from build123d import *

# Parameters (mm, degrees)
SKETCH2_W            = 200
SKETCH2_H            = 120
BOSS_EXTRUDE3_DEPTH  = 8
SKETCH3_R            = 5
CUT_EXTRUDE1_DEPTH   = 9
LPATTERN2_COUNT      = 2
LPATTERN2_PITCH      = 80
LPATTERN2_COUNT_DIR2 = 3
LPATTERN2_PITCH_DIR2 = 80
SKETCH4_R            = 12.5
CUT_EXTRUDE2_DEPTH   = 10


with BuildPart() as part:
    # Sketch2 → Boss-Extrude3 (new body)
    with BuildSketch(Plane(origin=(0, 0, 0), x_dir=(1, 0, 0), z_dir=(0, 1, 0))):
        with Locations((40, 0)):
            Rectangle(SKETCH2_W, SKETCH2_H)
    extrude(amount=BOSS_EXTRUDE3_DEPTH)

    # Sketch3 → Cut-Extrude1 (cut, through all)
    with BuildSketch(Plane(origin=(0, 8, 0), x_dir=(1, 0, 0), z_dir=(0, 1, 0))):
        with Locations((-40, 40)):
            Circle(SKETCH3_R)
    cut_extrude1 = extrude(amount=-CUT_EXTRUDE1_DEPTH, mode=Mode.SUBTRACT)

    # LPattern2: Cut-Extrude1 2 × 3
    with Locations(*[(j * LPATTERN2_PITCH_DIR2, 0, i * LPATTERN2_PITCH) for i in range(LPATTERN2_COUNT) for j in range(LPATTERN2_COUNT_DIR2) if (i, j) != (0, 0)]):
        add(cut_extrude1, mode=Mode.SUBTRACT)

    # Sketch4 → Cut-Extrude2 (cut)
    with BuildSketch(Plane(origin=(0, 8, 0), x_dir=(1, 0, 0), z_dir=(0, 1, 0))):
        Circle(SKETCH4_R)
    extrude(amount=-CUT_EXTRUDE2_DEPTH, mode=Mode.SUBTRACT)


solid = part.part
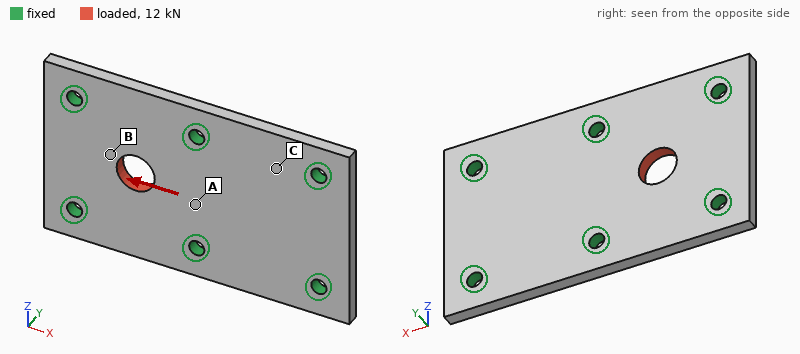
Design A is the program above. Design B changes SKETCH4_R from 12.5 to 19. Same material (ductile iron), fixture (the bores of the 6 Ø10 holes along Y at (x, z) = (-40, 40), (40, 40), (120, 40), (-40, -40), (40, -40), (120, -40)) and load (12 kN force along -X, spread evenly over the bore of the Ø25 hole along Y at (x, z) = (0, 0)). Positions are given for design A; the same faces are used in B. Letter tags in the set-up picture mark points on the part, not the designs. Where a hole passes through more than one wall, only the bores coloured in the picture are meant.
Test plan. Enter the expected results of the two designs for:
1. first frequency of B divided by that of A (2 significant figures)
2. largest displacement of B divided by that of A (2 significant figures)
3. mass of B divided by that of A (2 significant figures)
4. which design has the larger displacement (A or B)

1.0
0.90
0.97
A
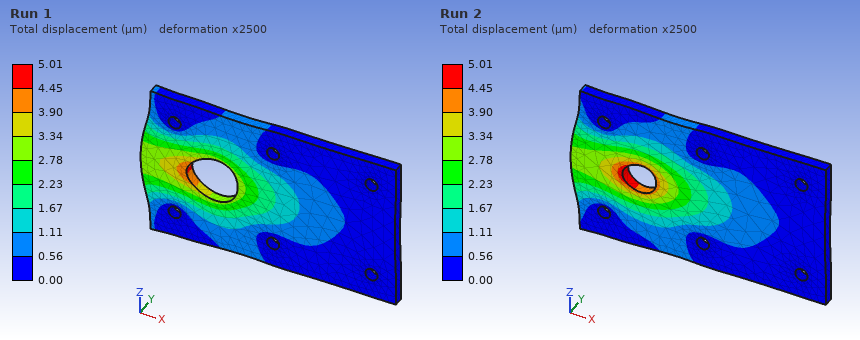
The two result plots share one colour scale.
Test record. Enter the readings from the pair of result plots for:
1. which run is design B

Run 1
